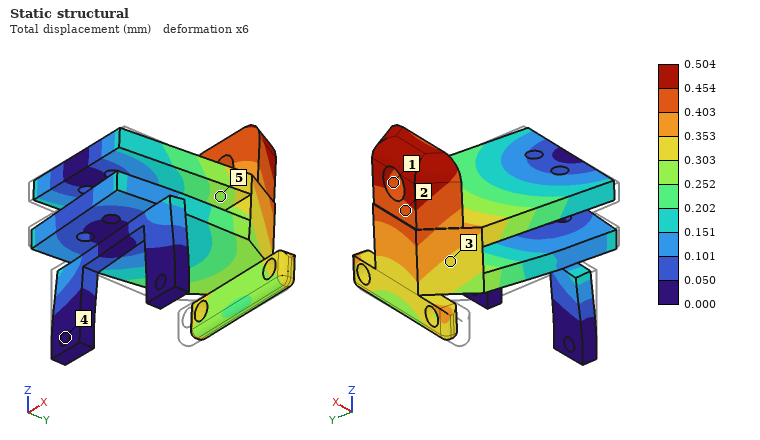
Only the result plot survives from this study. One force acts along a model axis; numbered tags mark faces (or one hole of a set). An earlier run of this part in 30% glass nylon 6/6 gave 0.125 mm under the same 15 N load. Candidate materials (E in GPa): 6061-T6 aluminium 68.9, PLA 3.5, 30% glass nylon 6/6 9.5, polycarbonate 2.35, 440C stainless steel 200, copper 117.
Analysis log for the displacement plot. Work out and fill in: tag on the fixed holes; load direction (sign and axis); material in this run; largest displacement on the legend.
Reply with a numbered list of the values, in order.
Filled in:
1. 4
2. +X
3. polycarbonate
4. 0.504 mm
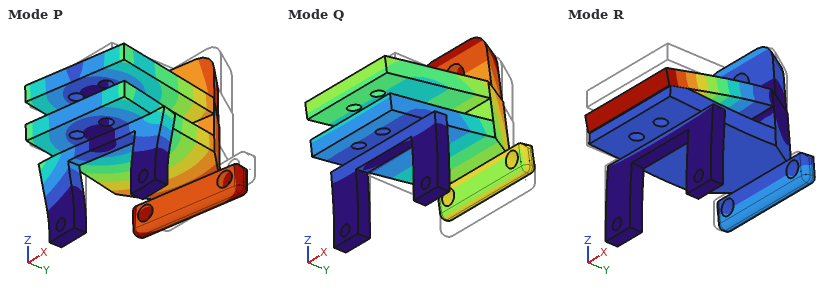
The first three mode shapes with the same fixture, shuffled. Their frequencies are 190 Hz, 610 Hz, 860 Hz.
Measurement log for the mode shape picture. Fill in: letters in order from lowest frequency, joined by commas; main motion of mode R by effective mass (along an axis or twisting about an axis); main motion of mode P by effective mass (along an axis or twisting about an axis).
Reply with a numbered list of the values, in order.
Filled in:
1. Q, P, R
2. along Z
3. along X
